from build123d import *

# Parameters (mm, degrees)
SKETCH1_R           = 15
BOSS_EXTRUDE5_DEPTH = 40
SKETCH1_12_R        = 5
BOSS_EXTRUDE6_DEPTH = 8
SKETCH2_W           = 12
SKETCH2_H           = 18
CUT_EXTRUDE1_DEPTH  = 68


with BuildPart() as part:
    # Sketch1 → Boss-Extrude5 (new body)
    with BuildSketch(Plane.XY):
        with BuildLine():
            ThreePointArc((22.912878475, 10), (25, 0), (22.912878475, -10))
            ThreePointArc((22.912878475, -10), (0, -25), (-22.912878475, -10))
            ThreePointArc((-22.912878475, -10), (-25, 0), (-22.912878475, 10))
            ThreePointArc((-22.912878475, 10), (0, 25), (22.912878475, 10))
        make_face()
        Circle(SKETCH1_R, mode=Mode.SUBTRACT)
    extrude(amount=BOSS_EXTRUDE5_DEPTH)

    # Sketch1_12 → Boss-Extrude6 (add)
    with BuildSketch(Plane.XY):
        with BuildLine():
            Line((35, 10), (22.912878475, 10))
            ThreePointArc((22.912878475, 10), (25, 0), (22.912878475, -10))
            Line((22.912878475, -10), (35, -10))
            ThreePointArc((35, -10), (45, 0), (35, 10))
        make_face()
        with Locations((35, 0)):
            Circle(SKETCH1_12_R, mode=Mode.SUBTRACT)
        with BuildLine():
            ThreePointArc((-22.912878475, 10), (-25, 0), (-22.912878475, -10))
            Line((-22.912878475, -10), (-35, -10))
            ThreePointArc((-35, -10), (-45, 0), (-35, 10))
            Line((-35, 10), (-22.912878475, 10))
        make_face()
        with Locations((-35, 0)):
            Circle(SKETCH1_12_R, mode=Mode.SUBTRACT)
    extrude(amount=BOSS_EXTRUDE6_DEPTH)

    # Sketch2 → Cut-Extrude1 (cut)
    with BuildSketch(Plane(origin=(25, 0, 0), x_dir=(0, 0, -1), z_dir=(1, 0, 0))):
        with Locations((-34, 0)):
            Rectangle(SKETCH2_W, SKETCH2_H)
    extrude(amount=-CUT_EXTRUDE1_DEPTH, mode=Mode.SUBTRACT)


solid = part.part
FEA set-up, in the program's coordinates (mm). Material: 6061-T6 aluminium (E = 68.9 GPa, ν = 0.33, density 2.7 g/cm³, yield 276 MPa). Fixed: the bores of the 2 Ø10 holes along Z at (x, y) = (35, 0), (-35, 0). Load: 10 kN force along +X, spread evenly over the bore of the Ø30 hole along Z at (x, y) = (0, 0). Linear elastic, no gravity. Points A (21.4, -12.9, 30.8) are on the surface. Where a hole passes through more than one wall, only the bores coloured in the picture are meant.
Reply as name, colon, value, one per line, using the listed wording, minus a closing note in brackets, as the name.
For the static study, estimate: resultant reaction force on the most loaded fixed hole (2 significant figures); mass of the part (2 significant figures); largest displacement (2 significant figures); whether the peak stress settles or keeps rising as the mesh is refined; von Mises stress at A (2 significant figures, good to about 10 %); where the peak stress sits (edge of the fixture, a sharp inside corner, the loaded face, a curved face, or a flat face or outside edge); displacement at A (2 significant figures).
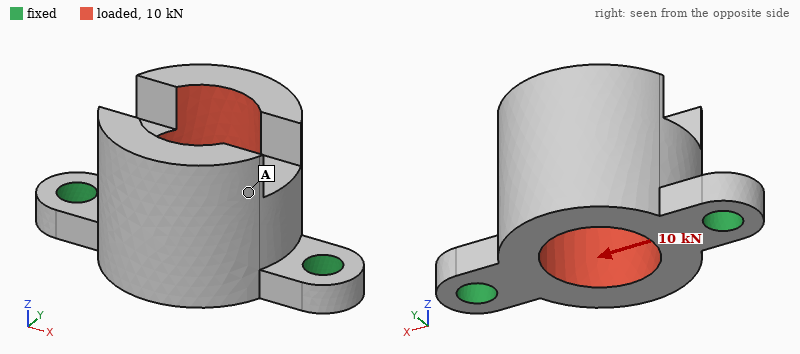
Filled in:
resultant reaction force on the most loaded fixed hole: 5.6 kN
mass of the part: 140 g
largest displacement: 33 µm
whether the peak stress settles or keeps rising as the mesh is refined: keeps rising
von Mises stress at A: 10 MPa
where the peak stress sits: edge of the fixture
displacement at A: 26 µm
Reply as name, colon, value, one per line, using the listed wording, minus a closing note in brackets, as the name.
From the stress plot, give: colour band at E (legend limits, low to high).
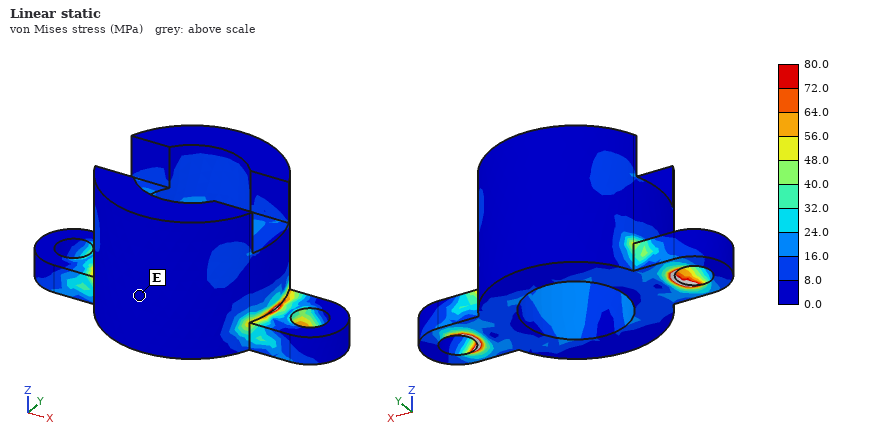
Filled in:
colour band at E: 0.0 to 8.0 MPa
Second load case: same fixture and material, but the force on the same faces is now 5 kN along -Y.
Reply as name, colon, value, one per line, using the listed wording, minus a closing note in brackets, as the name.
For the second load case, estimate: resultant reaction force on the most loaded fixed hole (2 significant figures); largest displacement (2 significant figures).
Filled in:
resultant reaction force on the most loaded fixed hole: 2.5 kN
largest displacement: 0.20 mm
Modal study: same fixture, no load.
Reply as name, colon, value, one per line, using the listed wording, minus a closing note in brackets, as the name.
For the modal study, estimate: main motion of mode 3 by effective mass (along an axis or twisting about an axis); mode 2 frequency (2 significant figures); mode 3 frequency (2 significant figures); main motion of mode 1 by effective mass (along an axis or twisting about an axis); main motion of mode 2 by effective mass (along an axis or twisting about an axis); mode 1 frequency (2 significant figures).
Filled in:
main motion of mode 3 by effective mass: along X
mode 2 frequency: 7300 Hz
mode 3 frequency: 9200 Hz
main motion of mode 1 by effective mass: along Y
main motion of mode 2 by effective mass: along Z
mode 1 frequency: 2400 Hz
